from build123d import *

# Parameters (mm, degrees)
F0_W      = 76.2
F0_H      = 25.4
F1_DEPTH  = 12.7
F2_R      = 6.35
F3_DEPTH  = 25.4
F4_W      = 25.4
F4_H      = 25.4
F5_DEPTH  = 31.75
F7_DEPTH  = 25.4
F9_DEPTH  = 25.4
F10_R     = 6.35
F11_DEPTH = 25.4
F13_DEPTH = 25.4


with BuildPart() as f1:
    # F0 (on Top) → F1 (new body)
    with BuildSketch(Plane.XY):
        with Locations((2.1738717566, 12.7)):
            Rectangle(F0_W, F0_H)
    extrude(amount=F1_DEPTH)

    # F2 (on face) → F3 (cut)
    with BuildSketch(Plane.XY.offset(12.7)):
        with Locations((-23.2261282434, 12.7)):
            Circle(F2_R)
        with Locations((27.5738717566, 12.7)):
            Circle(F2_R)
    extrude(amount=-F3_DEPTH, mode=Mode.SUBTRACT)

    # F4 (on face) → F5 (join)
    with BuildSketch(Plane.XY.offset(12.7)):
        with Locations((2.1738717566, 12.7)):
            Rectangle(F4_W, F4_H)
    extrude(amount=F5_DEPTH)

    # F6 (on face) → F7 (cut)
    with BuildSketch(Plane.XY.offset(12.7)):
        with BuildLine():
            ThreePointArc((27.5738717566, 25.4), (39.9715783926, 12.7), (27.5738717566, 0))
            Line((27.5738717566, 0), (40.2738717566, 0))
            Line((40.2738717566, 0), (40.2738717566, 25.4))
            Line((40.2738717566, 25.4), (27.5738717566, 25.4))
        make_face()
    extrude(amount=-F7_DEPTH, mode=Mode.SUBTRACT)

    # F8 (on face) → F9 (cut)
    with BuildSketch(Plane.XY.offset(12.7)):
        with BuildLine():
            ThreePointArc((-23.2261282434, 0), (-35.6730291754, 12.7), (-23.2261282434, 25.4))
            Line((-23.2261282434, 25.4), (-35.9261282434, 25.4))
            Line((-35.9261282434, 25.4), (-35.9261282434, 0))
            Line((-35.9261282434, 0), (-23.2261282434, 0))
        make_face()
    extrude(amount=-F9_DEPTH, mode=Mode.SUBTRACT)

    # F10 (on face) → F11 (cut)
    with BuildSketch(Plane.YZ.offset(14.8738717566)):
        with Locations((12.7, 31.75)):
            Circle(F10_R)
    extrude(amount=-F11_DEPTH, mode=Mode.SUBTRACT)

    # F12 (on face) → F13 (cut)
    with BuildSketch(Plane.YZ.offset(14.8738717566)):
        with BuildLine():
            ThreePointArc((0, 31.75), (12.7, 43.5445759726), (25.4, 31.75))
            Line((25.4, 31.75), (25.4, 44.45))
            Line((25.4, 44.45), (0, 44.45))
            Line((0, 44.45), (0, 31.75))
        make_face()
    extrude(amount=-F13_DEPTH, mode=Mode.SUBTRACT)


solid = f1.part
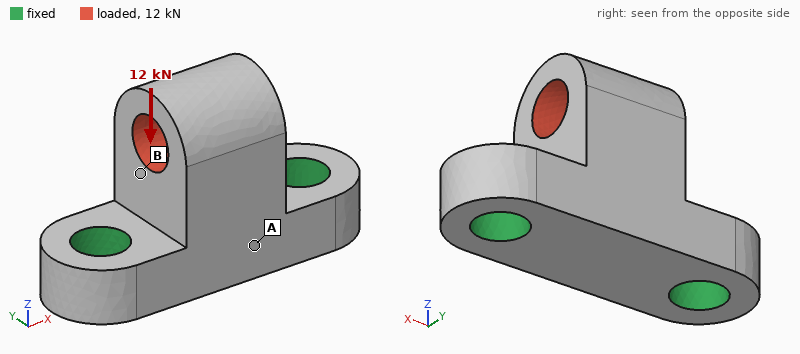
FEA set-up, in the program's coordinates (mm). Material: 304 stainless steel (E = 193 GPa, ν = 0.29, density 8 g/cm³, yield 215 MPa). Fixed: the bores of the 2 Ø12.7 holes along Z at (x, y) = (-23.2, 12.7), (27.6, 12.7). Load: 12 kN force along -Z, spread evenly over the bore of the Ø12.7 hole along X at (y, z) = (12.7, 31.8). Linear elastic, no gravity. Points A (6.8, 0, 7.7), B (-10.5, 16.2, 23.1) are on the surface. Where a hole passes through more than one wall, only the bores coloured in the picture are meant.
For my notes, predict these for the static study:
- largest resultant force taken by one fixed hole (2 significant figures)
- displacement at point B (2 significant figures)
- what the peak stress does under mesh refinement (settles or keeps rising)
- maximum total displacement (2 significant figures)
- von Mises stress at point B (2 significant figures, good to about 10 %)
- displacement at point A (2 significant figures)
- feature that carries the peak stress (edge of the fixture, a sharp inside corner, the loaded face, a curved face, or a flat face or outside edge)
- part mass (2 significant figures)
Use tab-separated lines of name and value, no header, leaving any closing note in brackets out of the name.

largest resultant force taken by one fixed hole	6.2 kN
displacement at point B	5.9 µm
what the peak stress does under mesh refinement	keeps rising
maximum total displacement	10 µm
von Mises stress at point B	23 MPa
displacement at point A	5.7 µm
feature that carries the peak stress	edge of the fixture
part mass	270 g
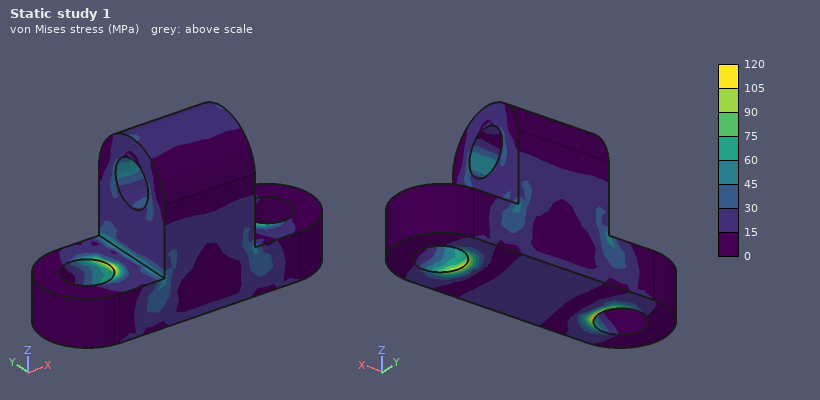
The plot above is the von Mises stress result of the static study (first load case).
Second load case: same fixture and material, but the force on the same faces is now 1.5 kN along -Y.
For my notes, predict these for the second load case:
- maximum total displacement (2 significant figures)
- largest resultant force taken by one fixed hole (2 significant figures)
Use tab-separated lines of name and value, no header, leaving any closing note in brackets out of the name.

maximum total displacement	11 µm
largest resultant force taken by one fixed hole	750 N
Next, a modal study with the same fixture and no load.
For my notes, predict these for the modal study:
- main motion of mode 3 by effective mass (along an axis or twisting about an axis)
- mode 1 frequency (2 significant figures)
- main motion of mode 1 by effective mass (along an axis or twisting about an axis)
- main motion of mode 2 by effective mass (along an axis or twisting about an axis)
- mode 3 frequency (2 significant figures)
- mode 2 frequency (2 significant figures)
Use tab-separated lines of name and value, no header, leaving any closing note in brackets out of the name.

main motion of mode 3 by effective mass	along Z
mode 1 frequency	7100 Hz
main motion of mode 1 by effective mass	along Y
main motion of mode 2 by effective mass	along X
mode 3 frequency	17 kHz
mode 2 frequency	12 kHz
